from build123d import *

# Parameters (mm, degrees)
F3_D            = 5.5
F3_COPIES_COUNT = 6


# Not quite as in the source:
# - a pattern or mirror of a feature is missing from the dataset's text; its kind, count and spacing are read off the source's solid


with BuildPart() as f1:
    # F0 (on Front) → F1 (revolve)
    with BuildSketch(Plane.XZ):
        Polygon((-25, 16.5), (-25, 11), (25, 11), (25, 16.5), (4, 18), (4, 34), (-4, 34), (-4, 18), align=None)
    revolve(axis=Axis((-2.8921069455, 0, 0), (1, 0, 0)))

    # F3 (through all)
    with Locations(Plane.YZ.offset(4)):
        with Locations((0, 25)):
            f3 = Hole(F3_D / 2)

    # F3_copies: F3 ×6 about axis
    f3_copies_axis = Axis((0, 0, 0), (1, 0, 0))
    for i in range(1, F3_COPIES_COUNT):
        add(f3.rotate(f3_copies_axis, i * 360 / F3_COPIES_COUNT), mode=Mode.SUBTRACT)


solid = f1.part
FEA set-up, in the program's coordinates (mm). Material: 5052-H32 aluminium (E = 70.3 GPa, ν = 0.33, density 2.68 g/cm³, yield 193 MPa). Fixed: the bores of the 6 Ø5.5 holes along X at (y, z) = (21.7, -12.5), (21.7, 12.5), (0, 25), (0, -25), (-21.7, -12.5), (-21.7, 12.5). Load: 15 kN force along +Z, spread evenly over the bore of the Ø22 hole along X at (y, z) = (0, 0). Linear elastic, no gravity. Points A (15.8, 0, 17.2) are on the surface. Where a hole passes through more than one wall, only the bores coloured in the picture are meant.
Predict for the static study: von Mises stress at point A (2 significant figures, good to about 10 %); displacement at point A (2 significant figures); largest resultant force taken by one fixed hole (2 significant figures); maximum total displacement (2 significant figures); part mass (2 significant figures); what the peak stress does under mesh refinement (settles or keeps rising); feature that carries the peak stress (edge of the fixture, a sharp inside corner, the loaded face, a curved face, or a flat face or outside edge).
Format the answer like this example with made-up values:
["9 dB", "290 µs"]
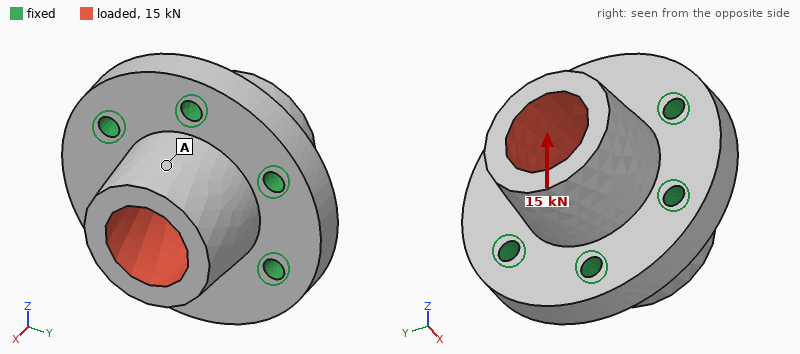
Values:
["7.1 MPa", "11 µm", "3.4 kN", "15 µm", "130 g", "keeps rising", "edge of the fixture"]
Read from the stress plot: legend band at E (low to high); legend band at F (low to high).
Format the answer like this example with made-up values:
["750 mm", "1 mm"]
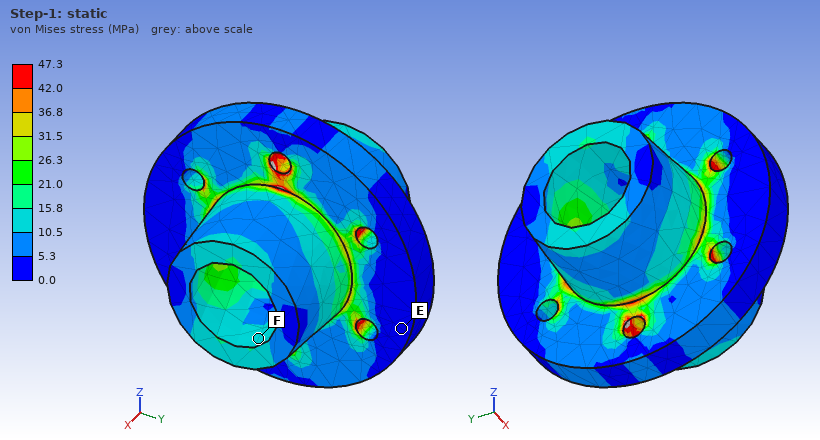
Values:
["0.0 to 5.3 MPa", "10.5 to 15.8 MPa"]
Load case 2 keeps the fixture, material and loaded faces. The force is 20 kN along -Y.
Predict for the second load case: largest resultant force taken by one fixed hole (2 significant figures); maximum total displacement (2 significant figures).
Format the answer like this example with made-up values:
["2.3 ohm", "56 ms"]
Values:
["4.1 kN", "20 µm"]
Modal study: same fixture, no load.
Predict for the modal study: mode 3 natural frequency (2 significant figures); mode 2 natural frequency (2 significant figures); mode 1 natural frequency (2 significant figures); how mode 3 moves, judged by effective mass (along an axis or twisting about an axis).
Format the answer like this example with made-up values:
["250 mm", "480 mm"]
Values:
["22 kHz", "18 kHz", "18 kHz", "along X"]
